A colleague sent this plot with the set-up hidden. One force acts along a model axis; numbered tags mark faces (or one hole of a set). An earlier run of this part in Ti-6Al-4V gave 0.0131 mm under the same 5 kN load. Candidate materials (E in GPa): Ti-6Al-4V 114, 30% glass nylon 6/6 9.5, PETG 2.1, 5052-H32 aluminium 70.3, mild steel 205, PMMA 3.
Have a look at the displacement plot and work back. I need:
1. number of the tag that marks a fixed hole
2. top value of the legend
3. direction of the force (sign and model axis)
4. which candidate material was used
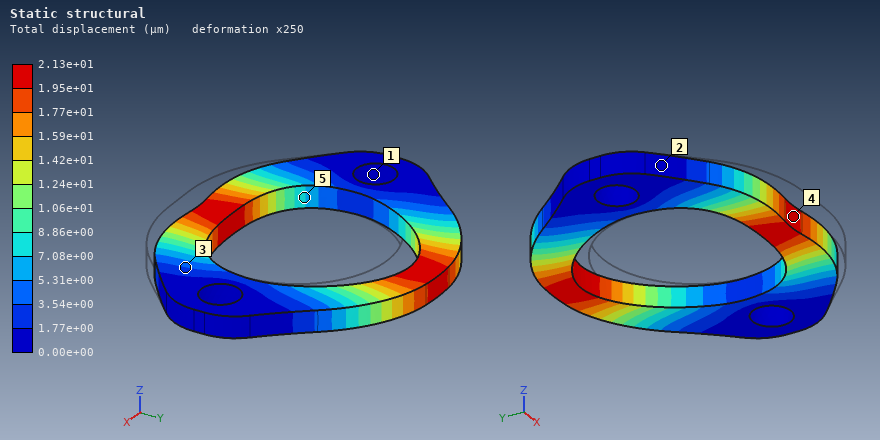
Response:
1
2.13e+01 µm
+Y
5052-H32 aluminium
